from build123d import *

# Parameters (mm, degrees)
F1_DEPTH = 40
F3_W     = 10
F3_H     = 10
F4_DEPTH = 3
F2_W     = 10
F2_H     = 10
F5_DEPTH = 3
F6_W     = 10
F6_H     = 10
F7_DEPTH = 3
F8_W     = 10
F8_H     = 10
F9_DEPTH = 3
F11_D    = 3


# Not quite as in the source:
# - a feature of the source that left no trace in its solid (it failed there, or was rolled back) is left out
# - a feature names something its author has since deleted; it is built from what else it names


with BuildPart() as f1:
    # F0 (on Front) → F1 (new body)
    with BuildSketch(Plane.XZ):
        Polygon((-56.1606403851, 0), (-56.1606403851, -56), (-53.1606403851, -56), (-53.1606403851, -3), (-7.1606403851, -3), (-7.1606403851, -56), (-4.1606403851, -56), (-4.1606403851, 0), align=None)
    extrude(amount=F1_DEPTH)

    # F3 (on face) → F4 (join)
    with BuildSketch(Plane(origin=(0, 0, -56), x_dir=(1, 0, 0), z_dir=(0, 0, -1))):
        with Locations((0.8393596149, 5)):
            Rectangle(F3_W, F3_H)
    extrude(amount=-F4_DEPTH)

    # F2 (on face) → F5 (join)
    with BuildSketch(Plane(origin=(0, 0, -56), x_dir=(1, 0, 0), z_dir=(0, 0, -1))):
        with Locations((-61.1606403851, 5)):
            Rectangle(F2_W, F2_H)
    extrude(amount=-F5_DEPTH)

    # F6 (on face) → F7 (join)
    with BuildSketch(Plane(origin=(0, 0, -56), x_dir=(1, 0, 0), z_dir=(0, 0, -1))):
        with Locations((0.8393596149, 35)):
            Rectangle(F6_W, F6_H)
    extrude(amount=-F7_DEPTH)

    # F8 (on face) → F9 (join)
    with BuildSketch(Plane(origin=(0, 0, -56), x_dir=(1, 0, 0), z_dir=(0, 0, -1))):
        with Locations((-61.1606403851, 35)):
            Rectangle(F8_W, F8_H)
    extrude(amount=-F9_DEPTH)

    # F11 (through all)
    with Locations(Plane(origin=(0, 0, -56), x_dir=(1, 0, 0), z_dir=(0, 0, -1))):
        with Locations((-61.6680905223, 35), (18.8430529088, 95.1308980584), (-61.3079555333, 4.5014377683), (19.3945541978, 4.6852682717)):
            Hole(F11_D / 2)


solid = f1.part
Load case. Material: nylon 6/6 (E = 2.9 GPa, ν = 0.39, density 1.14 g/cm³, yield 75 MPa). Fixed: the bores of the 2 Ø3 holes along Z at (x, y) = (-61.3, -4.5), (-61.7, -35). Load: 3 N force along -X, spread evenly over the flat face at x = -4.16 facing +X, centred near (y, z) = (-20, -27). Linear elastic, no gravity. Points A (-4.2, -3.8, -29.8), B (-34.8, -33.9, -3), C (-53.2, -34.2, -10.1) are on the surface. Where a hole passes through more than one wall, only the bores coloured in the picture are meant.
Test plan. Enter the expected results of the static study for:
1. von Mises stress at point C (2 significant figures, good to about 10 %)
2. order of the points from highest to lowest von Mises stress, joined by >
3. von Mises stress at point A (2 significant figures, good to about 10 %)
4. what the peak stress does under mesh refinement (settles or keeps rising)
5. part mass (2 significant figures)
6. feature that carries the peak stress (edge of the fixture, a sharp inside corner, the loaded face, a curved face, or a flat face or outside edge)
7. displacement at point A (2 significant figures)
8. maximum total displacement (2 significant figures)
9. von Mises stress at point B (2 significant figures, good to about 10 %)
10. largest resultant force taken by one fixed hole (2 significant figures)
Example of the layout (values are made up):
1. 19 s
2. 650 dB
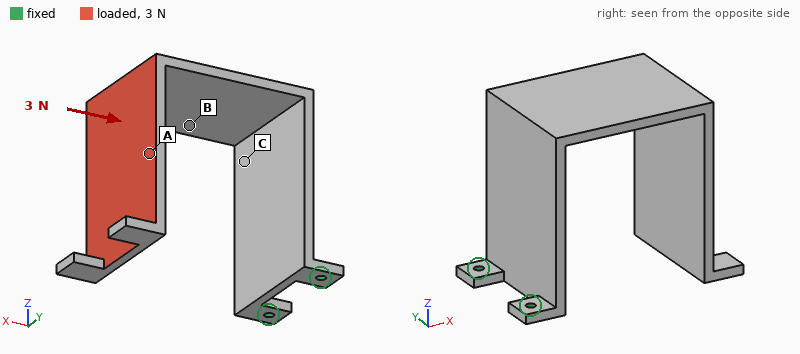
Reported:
1. 0.75 MPa
2. B > C > A
3. 0.29 MPa
4. keeps rising
5. 23 g
6. edge of the fixture
7. 0.67 mm
8. 1.0 mm
9. 1.3 MPa
10. 1.6 N
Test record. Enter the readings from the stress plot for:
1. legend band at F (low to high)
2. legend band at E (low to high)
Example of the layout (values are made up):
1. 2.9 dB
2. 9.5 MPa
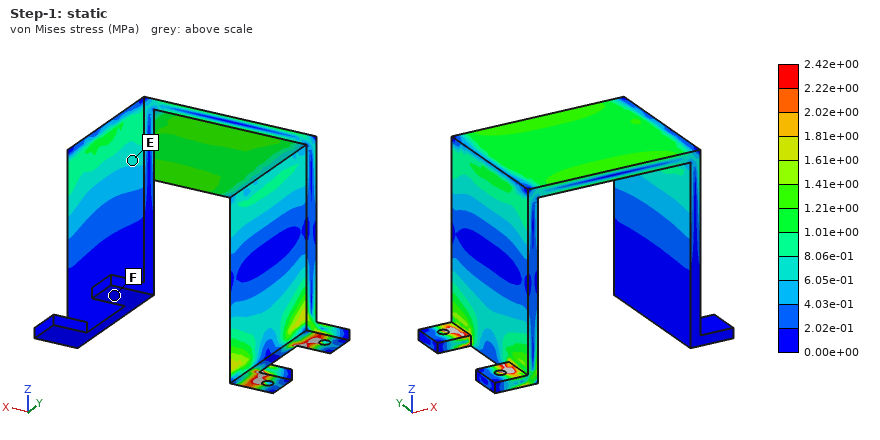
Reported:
1. 0.00e+00 to 2.02e-01 MPa
2. 6.05e-01 to 8.06e-01 MPa
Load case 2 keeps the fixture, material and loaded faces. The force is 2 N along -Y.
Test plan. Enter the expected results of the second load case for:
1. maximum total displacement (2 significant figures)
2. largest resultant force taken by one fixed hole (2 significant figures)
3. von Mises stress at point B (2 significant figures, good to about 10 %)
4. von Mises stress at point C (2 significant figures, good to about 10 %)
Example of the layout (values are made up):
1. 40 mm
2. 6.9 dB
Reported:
1. 1.1 mm
2. 3.9 N
3. 0.83 MPa
4. 1.4 MPa
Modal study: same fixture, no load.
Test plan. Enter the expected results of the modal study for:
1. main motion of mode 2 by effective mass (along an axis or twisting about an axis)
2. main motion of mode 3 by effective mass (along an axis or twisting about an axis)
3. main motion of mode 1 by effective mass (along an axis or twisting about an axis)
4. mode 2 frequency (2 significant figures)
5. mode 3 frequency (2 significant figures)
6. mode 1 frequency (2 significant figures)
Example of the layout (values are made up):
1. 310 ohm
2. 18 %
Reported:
1. along Y
2. along X
3. along Z
4. 78 Hz
5. 95 Hz
6. 49 Hz
